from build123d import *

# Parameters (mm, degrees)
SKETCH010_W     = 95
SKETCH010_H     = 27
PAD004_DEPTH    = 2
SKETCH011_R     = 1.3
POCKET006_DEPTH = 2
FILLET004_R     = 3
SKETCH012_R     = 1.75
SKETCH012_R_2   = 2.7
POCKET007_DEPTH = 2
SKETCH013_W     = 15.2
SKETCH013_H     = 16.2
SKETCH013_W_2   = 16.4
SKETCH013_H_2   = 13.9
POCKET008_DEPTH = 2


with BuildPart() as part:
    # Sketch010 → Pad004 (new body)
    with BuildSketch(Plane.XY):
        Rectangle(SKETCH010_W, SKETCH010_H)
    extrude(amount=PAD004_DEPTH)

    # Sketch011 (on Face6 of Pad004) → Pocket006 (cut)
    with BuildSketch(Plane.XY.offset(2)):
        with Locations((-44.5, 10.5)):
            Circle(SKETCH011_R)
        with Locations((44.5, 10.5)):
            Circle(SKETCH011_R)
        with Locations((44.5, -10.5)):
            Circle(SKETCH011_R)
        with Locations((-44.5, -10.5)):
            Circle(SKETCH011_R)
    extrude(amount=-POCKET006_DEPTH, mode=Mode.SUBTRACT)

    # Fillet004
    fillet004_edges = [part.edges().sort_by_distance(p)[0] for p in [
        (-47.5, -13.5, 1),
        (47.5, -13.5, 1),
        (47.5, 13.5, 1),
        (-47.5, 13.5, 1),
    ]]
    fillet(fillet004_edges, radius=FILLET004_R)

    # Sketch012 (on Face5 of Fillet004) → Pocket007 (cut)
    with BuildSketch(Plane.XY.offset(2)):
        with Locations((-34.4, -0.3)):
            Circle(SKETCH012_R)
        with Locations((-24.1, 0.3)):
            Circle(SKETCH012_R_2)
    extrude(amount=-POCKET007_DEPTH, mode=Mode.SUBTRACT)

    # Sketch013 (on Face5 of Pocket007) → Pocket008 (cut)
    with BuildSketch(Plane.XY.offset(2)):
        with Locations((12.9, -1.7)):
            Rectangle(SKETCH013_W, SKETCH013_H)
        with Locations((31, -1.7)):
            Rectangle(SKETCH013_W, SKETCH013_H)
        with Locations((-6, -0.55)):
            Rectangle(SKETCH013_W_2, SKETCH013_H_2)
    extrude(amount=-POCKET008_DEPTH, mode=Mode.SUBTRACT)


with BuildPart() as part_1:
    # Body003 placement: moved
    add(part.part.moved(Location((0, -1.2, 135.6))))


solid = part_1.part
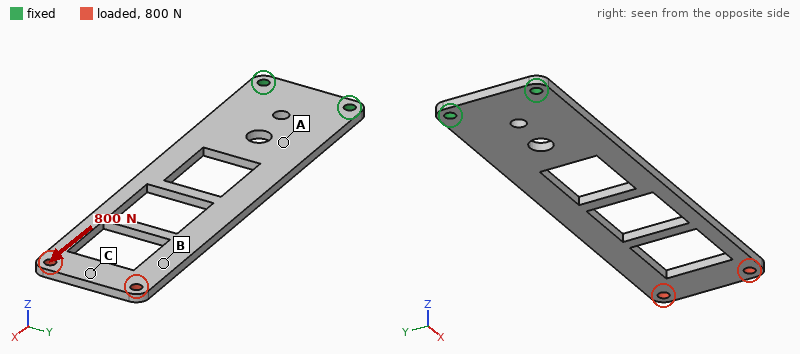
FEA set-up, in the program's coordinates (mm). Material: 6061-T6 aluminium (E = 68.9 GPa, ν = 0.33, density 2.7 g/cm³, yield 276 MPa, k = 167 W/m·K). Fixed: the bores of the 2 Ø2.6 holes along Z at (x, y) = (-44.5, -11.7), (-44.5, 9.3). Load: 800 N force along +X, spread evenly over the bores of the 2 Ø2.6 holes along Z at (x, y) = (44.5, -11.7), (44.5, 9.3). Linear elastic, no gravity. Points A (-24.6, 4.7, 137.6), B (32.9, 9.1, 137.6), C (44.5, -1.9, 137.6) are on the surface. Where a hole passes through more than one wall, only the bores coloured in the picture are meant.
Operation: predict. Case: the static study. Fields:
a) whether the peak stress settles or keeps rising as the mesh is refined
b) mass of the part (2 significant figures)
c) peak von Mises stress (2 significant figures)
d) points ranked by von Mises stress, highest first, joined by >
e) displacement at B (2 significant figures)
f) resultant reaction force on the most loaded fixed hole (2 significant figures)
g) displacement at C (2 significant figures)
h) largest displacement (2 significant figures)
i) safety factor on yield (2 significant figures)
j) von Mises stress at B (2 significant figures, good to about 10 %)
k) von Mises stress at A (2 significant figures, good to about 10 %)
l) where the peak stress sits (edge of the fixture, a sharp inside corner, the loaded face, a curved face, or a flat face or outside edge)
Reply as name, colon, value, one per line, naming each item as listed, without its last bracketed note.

whether the peak stress settles or keeps rising as the mesh is refined: settles
mass of the part: 9.6 g
peak von Mises stress: 90 MPa
points ranked by von Mises stress, highest first, joined by >: B > A > C
displacement at B: 35 µm
resultant reaction force on the most loaded fixed hole: 410 N
displacement at C: 48 µm
largest displacement: 56 µm
safety factor on yield: 3.1
von Mises stress at B: 30 MPa
von Mises stress at A: 16 MPa
where the peak stress sits: the loaded face
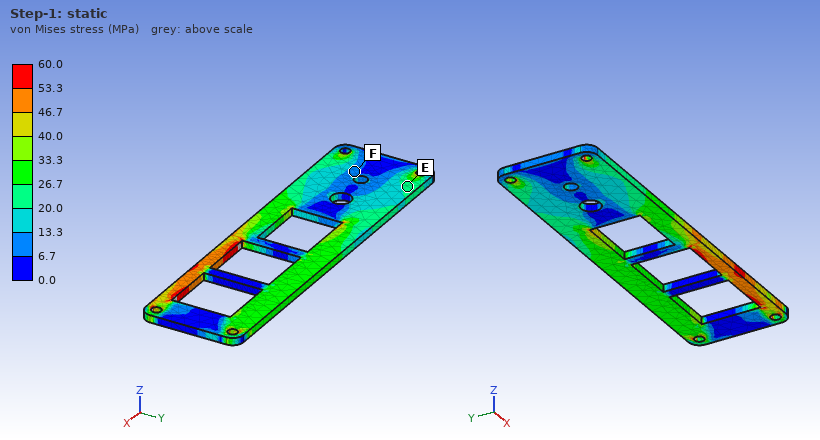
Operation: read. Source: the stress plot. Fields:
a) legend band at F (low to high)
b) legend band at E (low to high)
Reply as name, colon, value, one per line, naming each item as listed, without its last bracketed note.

legend band at F: 6.7 to 13.3 MPa
legend band at E: 20.0 to 26.7 MPa
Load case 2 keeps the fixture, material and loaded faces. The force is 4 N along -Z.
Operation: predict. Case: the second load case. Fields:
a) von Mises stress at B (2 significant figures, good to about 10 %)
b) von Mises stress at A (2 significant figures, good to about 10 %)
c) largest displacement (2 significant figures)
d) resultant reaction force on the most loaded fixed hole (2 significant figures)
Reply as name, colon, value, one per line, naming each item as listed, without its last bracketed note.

von Mises stress at B: 6.6 MPa
von Mises stress at A: 19 MPa
largest displacement: 1.2 mm
resultant reaction force on the most loaded fixed hole: 2.0 N
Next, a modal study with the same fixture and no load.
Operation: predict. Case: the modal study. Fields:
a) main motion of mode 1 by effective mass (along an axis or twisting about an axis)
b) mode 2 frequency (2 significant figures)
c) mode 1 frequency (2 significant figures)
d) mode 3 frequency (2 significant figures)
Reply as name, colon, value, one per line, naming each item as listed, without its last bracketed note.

main motion of mode 1 by effective mass: along Z
mode 2 frequency: 1100 Hz
mode 1 frequency: 210 Hz
mode 3 frequency: 1100 Hz
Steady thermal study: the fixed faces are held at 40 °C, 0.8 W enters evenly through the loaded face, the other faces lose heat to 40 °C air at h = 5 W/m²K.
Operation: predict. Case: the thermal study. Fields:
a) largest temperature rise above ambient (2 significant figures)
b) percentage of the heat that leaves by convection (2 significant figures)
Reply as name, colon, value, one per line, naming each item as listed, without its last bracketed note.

largest temperature rise above ambient: 14 K
percentage of the heat that leaves by convection: 15 %
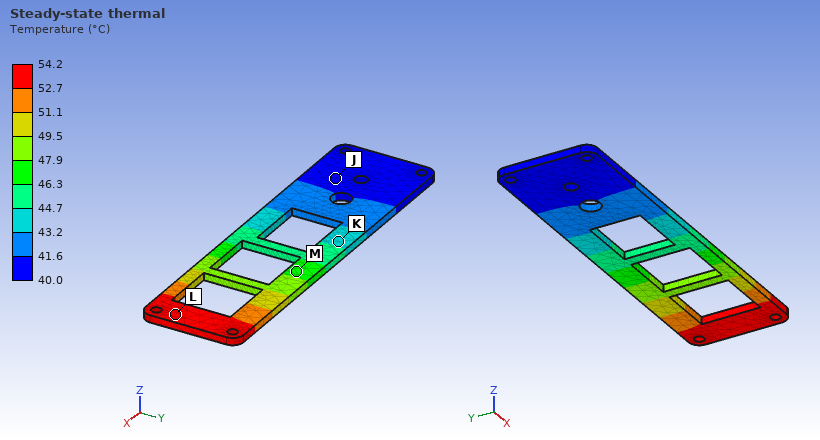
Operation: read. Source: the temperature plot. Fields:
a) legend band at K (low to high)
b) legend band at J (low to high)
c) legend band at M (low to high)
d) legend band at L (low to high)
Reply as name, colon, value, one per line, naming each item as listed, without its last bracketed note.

legend band at K: 43.2 to 44.7 °C
legend band at J: 40.0 to 41.6 °C
legend band at M: 46.3 to 47.9 °C
legend band at L: 52.7 to 54.2 °C
